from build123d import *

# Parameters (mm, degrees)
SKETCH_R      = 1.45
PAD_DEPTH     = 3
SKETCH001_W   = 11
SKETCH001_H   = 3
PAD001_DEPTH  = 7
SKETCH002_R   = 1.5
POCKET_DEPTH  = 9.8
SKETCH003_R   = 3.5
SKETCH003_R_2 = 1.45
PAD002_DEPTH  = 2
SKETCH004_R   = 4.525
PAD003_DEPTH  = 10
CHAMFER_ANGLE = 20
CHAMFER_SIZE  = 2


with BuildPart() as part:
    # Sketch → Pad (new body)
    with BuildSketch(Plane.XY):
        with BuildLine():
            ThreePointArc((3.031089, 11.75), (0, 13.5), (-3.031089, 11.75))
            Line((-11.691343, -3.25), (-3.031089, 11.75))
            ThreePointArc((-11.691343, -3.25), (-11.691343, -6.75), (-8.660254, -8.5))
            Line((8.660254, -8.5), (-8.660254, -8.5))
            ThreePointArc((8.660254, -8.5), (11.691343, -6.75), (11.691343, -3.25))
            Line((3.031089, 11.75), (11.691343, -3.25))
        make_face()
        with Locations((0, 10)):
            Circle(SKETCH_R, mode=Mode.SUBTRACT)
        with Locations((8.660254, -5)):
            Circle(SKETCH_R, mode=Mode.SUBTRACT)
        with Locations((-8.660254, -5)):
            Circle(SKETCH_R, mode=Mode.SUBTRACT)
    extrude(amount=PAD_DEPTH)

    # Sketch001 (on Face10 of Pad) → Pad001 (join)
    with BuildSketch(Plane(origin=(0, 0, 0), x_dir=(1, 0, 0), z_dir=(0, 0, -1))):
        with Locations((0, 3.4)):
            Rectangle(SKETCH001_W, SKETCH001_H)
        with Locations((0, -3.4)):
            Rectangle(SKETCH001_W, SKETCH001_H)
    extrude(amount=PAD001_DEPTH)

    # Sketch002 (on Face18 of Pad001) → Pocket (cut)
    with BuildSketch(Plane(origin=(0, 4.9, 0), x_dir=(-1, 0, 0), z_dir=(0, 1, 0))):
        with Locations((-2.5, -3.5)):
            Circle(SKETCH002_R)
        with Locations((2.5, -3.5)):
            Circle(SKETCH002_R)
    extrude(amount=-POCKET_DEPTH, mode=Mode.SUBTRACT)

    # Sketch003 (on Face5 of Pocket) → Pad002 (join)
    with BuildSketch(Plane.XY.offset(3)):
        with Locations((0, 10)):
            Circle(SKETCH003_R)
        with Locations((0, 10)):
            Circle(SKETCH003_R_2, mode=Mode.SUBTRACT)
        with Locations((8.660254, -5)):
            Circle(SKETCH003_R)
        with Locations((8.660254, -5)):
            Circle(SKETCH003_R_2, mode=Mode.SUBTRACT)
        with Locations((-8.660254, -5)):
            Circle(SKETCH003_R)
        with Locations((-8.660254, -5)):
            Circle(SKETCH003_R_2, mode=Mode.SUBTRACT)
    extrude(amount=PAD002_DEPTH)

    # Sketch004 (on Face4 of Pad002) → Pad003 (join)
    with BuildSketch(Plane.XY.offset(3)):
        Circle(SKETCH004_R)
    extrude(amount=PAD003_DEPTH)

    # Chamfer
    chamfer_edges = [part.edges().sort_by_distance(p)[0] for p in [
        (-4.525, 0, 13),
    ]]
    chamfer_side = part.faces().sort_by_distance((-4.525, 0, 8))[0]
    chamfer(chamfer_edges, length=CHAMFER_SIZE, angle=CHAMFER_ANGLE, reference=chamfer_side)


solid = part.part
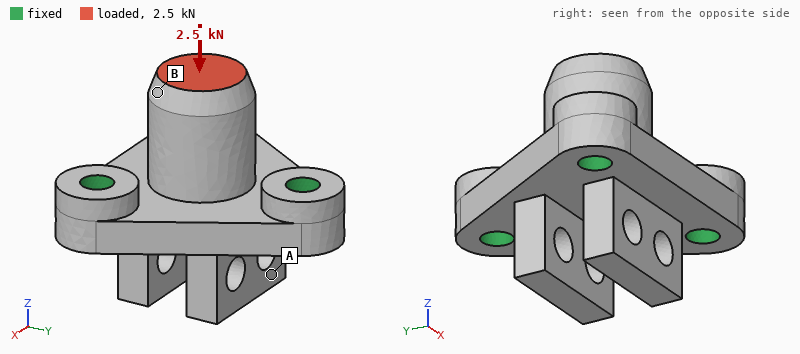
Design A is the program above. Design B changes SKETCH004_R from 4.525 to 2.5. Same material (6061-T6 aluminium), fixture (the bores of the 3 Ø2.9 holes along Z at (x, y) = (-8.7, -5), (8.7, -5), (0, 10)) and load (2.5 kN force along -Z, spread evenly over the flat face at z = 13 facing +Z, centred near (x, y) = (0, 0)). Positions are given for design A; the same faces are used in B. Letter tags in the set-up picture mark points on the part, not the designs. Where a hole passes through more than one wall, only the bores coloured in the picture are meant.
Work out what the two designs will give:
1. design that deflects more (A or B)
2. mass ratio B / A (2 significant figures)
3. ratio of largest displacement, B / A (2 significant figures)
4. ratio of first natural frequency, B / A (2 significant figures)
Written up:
B
0.80
2.3
0.95
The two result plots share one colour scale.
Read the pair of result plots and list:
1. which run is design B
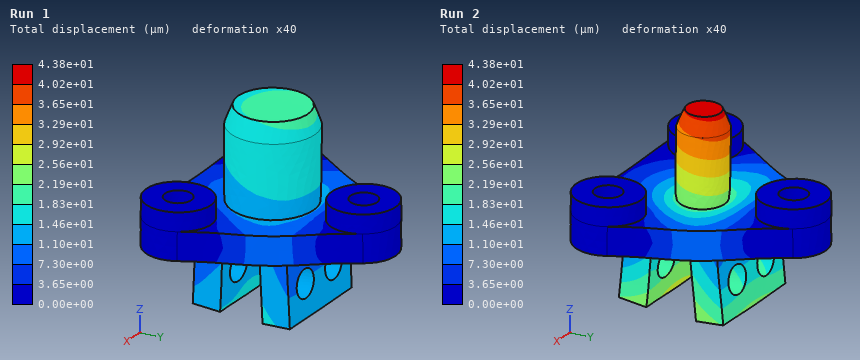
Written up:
Run 2
